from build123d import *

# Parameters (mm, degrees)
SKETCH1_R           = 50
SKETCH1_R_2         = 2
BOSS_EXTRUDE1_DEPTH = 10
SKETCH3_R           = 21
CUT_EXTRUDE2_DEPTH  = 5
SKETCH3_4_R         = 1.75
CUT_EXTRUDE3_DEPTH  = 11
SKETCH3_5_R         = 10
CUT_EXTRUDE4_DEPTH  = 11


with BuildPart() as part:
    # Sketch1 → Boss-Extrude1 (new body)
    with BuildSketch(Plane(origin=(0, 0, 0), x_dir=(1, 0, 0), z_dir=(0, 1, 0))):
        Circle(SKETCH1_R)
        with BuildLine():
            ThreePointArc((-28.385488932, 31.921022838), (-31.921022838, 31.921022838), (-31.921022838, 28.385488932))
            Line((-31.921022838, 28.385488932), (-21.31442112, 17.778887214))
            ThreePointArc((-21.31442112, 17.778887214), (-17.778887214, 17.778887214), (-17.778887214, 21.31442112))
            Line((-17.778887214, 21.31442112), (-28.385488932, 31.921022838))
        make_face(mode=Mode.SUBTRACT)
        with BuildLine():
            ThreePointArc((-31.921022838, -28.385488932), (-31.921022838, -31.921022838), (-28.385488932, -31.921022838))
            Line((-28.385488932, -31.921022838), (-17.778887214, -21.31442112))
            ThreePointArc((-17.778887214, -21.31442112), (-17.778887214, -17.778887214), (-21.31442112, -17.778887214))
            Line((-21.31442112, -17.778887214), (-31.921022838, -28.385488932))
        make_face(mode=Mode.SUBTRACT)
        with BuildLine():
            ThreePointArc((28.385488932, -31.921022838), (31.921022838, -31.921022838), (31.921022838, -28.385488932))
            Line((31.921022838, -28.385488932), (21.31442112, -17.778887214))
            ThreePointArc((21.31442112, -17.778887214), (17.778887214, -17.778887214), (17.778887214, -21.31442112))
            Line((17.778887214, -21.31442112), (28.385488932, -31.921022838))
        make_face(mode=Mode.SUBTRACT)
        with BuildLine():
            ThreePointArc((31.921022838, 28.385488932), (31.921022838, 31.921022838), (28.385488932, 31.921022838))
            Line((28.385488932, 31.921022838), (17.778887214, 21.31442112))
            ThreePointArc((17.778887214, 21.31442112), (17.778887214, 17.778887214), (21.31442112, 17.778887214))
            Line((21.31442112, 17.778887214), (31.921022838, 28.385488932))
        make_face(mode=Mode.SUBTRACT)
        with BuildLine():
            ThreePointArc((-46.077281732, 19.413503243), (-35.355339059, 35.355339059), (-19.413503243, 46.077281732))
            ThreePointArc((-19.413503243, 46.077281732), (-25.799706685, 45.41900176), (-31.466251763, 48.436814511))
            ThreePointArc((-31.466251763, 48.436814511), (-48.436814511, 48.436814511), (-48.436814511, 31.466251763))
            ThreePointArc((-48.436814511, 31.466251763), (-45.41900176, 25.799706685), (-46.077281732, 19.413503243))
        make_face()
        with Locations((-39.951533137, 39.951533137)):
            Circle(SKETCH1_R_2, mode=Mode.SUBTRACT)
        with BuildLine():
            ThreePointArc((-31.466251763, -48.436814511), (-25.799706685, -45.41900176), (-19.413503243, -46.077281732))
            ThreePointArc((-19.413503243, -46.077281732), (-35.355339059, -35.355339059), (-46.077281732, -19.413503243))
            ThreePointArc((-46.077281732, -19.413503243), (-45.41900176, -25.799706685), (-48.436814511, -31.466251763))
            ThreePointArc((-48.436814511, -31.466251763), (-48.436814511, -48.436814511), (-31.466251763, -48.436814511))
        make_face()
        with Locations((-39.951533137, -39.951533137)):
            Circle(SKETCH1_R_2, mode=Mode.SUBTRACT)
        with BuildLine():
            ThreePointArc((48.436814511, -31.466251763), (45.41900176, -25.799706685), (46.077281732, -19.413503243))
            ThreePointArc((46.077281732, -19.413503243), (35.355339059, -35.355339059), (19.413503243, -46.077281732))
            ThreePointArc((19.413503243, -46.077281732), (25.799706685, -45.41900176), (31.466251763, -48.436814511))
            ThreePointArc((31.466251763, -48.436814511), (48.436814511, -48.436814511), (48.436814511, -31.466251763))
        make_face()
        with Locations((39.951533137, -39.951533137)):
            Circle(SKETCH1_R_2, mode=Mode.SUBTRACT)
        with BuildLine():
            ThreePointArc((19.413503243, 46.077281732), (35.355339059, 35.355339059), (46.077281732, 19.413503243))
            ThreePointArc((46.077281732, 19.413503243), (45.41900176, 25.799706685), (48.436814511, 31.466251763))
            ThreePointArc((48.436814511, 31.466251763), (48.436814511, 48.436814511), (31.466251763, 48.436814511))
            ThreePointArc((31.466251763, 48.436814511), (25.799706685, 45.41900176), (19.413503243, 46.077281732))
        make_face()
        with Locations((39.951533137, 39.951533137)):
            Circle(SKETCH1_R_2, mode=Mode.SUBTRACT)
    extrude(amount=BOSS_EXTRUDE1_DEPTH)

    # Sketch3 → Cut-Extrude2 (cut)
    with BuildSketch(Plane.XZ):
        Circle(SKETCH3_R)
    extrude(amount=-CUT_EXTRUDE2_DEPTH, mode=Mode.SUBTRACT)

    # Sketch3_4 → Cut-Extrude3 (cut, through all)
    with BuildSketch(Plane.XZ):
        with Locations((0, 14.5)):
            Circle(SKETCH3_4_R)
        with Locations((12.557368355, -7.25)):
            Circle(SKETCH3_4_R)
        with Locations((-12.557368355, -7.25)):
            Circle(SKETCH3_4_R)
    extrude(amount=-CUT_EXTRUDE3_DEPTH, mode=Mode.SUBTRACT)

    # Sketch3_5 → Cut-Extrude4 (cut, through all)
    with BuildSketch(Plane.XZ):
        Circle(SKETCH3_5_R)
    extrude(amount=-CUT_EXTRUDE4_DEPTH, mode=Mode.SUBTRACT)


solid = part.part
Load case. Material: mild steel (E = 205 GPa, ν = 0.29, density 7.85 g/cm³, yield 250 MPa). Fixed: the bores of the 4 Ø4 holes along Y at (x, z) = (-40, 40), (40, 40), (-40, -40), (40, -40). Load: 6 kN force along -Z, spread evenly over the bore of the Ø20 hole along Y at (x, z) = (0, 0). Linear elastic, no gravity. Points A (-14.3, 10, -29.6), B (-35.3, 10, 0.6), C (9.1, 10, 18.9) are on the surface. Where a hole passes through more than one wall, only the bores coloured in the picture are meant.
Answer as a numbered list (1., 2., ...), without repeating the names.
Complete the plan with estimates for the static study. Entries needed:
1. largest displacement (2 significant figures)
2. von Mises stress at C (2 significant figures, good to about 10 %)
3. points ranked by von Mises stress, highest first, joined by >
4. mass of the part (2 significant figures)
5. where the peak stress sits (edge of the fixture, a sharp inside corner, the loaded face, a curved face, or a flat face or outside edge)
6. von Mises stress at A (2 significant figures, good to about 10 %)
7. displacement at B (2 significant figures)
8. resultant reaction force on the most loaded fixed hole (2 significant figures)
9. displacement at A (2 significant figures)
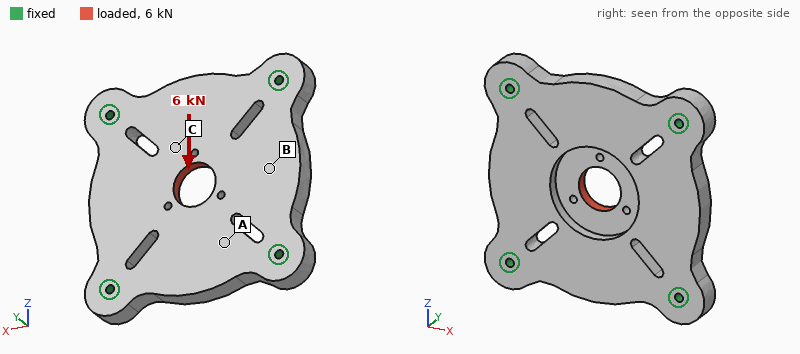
1. 4.3 µm
2. 15 MPa
3. C > A > B
4. 650 g
5. a curved face
6. 8.0 MPa
7. 0.95 µm
8. 1.7 kN
9. 2.3 µm
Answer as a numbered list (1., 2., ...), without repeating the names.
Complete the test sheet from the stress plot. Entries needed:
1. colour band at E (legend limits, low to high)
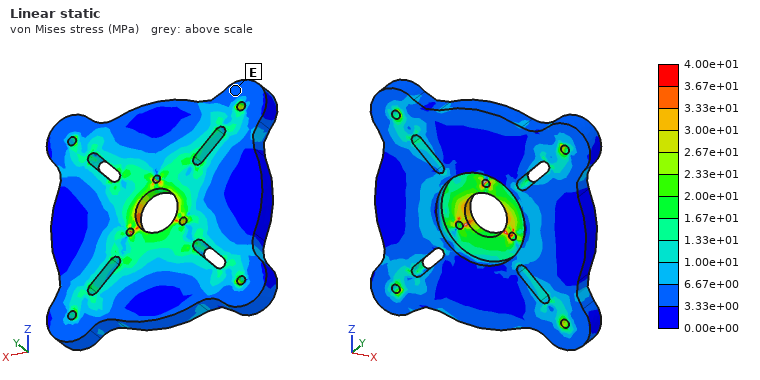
1. 3.33e+00 to 6.67e+00 MPa
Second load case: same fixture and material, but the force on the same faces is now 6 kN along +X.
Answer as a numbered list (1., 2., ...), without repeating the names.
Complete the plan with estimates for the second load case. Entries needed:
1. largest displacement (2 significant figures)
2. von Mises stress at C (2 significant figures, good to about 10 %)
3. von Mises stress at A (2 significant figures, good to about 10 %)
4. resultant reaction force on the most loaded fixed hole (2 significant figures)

1. 4.1 µm
2. 12 MPa
3. 6.5 MPa
4. 1.7 kN
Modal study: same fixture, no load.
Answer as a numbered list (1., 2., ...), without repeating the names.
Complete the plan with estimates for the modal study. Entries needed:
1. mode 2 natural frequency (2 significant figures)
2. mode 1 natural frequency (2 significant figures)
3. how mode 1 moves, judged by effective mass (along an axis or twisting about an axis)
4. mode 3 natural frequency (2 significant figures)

1. 7100 Hz
2. 4800 Hz
3. along Y
4. 7100 Hz
